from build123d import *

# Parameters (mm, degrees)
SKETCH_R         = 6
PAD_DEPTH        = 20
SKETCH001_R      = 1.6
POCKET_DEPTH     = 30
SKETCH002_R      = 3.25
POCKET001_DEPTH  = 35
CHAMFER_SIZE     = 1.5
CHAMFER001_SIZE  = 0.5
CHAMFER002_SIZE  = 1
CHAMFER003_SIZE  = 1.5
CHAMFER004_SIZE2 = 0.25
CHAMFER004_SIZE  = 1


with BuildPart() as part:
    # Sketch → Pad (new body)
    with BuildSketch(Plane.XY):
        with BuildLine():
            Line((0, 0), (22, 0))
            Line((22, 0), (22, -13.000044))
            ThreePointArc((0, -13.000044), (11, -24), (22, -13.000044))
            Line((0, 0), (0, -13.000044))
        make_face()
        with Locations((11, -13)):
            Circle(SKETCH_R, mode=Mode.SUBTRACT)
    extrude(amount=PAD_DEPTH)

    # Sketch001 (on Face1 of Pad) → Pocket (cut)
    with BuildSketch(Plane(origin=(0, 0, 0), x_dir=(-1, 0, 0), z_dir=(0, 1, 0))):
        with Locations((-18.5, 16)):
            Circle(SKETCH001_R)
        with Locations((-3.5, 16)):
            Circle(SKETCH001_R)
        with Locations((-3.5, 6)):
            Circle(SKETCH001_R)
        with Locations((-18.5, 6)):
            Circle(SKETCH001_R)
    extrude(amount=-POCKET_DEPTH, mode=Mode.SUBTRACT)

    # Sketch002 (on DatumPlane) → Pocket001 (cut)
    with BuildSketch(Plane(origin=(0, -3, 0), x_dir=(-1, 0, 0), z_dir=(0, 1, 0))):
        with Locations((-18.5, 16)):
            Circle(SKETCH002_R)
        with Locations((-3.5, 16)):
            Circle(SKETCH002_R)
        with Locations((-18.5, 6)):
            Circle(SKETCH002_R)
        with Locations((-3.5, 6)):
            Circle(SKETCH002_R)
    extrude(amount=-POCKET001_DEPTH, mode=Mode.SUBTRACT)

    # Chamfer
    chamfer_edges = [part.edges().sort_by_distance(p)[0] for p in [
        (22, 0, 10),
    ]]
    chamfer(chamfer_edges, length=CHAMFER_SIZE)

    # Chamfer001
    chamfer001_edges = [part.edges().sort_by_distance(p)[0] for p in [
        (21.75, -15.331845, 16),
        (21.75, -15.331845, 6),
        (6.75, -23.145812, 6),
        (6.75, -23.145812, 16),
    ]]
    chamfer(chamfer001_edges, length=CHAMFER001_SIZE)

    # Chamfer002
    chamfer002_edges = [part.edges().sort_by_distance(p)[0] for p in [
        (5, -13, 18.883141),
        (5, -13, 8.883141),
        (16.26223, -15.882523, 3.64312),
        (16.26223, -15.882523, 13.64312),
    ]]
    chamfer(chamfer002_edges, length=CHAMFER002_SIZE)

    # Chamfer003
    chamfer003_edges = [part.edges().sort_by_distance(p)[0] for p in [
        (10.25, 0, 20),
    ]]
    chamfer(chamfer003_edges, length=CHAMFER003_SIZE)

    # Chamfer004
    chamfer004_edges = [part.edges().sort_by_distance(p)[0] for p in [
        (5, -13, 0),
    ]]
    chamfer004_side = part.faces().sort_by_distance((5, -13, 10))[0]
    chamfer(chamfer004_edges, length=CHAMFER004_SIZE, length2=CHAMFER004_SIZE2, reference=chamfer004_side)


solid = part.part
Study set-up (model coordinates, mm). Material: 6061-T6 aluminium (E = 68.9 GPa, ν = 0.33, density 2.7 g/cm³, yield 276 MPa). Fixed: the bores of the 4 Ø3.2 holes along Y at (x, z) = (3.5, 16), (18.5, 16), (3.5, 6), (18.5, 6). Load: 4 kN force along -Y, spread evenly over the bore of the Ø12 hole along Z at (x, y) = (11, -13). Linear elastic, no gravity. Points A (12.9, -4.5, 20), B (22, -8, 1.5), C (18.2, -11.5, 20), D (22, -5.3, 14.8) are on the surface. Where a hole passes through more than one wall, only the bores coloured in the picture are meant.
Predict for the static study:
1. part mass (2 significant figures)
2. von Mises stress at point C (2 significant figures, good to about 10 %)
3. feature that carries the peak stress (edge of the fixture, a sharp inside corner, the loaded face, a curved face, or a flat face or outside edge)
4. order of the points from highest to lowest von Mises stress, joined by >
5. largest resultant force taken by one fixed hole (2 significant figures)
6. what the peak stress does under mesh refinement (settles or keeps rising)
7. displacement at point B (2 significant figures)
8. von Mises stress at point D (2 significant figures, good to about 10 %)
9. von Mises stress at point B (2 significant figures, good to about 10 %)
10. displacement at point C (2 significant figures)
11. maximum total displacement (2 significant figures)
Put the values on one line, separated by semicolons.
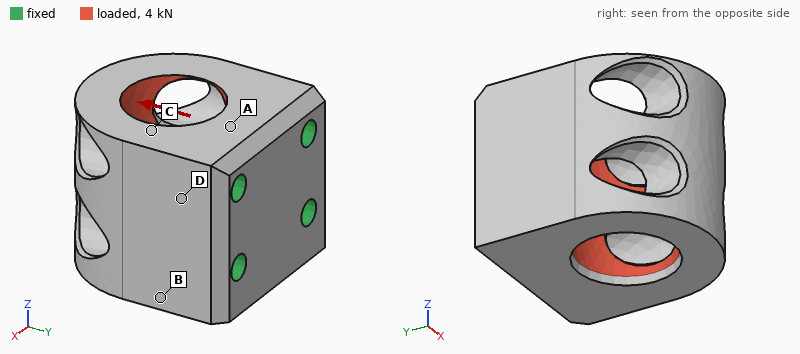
13 g; 67 MPa; a sharp inside corner; C > D > B > A; 1.1 kN; keeps rising; 6.6 µm; 39 MPa; 21 MPa; 7.9 µm; 20 µm
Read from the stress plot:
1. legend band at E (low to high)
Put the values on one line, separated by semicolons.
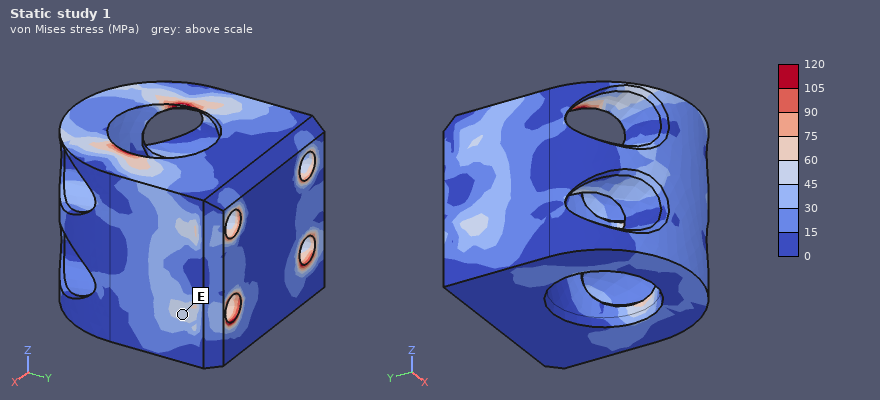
45 to 60 MPa
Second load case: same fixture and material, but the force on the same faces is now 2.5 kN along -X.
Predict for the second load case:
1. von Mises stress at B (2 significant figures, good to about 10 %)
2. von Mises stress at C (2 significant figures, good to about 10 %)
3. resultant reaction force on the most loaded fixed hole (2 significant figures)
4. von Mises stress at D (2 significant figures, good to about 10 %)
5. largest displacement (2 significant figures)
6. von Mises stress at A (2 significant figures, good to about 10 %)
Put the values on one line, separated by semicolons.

41 MPa; 60 MPa; 1.2 kN; 52 MPa; 38 µm; 33 MPa
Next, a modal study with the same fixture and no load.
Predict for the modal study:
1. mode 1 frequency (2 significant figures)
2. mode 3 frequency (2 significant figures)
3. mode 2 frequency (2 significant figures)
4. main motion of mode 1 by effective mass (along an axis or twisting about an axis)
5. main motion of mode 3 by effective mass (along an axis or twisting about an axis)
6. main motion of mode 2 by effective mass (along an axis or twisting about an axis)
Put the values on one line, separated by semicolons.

11 kHz; 23 kHz; 15 kHz; along Z; twisting about Y; along X
